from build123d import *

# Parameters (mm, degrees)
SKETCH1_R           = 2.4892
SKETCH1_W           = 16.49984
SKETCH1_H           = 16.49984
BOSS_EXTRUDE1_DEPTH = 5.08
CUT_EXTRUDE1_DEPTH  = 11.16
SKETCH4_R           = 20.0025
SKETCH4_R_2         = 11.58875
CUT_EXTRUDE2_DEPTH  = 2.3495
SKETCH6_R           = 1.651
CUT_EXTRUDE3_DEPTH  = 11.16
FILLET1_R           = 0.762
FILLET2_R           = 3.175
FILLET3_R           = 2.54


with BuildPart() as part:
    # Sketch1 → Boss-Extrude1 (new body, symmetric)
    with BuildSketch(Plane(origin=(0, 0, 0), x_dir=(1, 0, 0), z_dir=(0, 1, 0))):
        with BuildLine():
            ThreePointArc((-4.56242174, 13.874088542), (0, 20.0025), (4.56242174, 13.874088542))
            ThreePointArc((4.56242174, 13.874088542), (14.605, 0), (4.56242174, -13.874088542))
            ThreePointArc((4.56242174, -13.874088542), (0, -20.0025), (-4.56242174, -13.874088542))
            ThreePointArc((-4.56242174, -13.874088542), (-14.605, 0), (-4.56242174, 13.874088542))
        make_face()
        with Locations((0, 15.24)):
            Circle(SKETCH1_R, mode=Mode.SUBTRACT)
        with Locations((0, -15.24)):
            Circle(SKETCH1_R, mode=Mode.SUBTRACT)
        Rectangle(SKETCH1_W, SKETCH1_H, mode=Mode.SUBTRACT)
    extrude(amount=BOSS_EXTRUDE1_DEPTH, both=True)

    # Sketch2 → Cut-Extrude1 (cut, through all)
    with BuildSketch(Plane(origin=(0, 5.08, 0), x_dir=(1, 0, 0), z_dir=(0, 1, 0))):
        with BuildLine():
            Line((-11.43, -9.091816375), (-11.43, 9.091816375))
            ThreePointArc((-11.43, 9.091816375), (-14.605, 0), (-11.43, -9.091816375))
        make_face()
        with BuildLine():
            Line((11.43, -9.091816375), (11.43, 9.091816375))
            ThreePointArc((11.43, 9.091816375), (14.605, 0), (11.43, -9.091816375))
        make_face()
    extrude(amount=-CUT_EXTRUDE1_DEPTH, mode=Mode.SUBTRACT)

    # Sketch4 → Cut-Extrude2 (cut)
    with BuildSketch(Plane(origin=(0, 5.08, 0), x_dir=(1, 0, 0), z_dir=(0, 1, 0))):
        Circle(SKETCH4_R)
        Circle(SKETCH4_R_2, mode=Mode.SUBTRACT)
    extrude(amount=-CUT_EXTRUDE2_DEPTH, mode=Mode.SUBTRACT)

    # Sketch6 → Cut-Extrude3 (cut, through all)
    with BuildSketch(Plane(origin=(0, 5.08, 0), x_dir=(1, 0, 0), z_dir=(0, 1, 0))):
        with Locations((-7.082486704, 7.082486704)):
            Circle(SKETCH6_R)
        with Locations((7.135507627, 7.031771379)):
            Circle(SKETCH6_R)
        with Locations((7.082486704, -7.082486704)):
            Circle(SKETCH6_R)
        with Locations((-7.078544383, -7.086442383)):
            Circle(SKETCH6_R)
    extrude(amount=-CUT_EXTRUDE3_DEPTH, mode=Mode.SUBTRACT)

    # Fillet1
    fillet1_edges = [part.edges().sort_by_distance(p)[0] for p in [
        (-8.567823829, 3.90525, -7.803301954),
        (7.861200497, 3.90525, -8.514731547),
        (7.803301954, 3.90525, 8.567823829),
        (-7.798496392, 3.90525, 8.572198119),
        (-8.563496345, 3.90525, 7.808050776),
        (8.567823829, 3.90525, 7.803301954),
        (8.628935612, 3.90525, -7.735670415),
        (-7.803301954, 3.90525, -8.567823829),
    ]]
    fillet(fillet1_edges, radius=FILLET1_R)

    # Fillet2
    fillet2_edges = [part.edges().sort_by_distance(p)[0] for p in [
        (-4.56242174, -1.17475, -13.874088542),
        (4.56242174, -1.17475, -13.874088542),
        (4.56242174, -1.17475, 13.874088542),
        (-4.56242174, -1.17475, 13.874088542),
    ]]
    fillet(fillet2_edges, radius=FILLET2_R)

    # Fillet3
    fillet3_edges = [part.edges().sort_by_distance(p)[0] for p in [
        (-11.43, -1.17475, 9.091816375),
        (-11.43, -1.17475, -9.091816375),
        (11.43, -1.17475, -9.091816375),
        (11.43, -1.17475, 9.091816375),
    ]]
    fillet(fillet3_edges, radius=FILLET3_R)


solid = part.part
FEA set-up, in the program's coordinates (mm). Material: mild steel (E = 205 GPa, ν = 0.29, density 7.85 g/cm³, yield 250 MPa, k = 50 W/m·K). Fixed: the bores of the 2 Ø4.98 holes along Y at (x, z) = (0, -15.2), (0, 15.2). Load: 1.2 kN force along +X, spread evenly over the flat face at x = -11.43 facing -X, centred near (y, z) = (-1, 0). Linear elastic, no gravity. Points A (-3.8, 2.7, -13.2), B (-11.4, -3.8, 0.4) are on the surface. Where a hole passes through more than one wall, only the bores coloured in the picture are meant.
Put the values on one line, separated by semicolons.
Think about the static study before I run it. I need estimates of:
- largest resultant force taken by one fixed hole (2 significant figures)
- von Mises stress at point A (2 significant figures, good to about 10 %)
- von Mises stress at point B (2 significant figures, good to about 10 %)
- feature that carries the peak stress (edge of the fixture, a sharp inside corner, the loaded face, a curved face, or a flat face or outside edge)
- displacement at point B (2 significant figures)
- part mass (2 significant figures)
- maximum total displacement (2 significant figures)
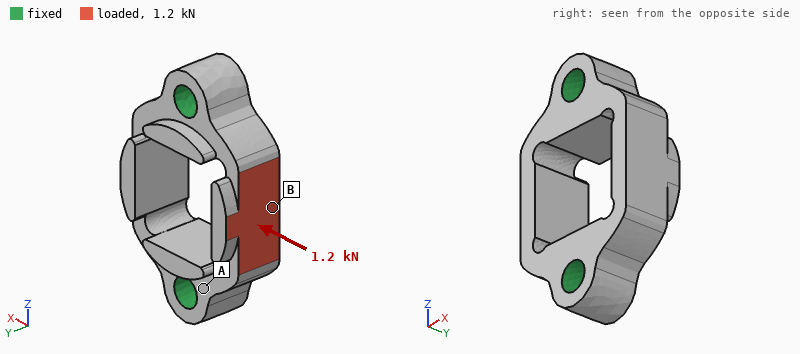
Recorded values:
760 N; 19 MPa; 120 MPa; a curved face; 11 µm; 25 g; 13 µm
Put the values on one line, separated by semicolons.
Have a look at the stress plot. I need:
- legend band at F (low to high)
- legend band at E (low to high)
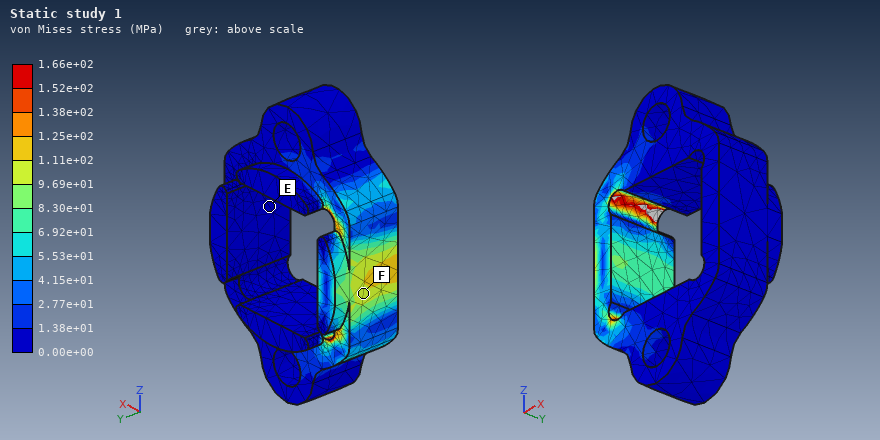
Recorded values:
9.69e+01 to 1.11e+02 MPa; 0.00e+00 to 1.38e+01 MPa
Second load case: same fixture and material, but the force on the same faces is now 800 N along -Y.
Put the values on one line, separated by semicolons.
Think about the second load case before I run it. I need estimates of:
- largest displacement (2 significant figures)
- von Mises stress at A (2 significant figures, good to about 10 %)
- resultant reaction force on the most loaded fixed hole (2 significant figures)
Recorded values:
11 µm; 60 MPa; 400 N
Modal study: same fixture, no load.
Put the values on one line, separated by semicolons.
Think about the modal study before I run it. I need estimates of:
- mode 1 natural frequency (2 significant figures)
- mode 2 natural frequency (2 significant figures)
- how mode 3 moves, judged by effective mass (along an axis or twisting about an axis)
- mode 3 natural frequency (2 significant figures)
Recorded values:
25 kHz; 27 kHz; along X; 28 kHz
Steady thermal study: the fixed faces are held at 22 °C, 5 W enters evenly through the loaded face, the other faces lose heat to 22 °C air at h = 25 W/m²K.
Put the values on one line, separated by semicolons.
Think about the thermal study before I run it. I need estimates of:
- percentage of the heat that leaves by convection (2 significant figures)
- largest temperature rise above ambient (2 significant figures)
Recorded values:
4.6 %; 23 K
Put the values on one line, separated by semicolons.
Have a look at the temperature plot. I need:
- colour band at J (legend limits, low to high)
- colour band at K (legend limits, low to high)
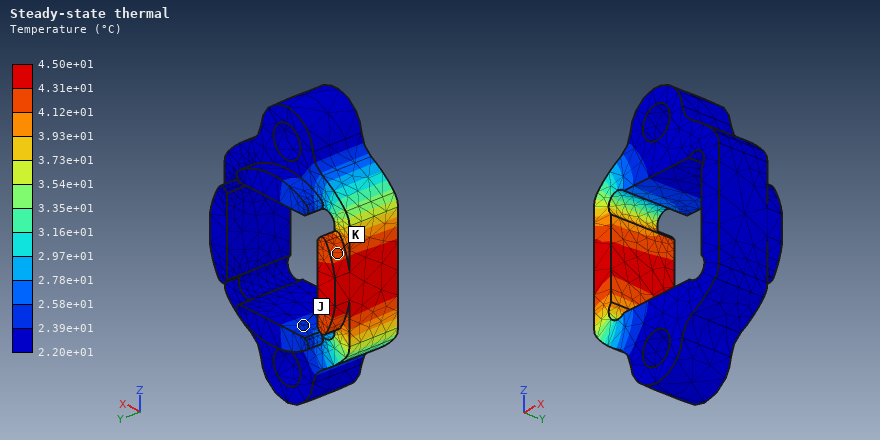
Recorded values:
2.39e+01 to 2.58e+01 °C; 4.12e+01 to 4.31e+01 °C
